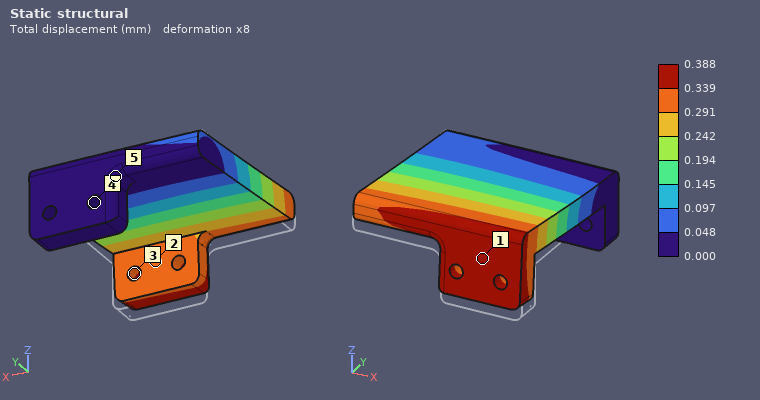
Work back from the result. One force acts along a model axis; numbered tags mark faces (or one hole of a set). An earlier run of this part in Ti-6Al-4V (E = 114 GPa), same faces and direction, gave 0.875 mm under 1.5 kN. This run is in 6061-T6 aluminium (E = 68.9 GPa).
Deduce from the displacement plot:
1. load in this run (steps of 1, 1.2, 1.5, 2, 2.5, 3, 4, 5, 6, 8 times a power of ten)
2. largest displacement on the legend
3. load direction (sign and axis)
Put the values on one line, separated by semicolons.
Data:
400 N; 0.388 mm; +Z
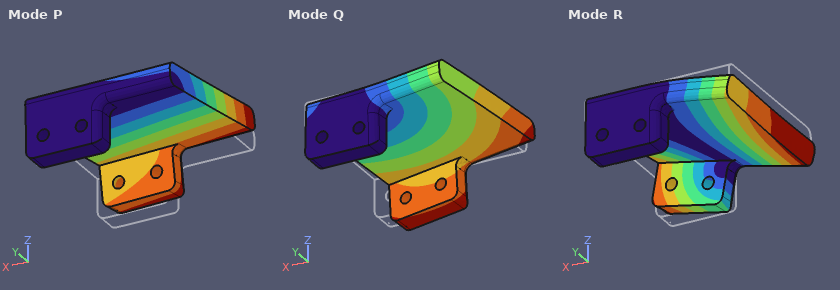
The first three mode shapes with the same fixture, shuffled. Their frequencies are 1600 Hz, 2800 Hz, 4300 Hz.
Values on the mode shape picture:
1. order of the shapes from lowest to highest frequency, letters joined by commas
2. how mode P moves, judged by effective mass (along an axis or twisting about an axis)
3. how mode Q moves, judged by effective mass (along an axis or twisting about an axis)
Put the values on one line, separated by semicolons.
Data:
P, Q, R; along Z; along X
